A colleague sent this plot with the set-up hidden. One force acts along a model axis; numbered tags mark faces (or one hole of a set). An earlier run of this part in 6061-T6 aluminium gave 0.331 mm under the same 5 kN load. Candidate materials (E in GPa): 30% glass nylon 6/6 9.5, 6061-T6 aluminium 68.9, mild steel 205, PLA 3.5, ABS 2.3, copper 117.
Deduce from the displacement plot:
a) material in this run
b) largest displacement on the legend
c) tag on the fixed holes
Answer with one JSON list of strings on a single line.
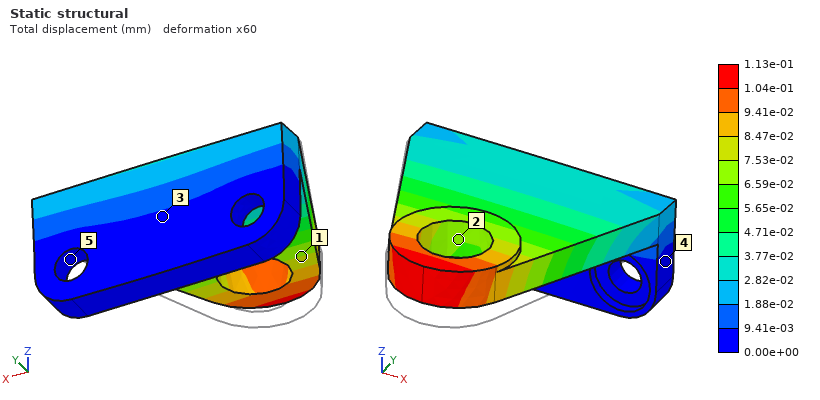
["mild steel", "1.13e-01 mm", "5"]
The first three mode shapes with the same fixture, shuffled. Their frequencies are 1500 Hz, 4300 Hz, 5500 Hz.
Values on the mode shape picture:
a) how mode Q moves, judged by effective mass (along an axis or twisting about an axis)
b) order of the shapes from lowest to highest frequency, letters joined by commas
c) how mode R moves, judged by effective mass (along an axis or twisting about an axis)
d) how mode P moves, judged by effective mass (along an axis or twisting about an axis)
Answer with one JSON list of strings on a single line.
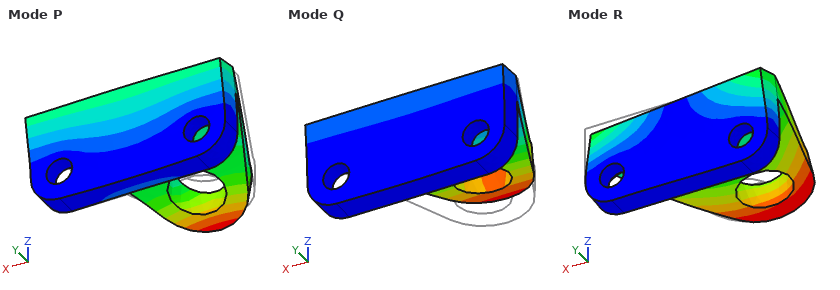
["along Z", "Q, R, P", "along X", "along Y"]
